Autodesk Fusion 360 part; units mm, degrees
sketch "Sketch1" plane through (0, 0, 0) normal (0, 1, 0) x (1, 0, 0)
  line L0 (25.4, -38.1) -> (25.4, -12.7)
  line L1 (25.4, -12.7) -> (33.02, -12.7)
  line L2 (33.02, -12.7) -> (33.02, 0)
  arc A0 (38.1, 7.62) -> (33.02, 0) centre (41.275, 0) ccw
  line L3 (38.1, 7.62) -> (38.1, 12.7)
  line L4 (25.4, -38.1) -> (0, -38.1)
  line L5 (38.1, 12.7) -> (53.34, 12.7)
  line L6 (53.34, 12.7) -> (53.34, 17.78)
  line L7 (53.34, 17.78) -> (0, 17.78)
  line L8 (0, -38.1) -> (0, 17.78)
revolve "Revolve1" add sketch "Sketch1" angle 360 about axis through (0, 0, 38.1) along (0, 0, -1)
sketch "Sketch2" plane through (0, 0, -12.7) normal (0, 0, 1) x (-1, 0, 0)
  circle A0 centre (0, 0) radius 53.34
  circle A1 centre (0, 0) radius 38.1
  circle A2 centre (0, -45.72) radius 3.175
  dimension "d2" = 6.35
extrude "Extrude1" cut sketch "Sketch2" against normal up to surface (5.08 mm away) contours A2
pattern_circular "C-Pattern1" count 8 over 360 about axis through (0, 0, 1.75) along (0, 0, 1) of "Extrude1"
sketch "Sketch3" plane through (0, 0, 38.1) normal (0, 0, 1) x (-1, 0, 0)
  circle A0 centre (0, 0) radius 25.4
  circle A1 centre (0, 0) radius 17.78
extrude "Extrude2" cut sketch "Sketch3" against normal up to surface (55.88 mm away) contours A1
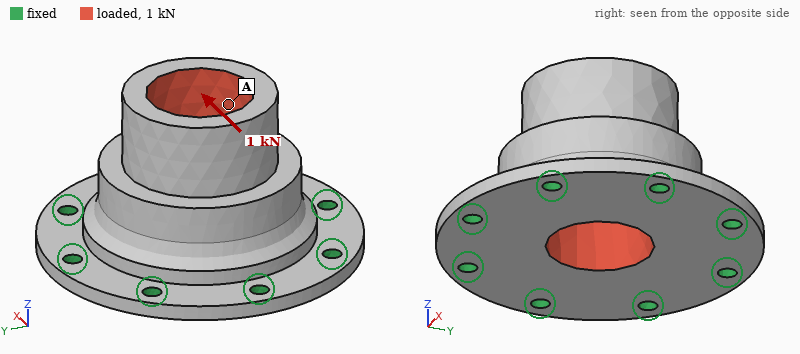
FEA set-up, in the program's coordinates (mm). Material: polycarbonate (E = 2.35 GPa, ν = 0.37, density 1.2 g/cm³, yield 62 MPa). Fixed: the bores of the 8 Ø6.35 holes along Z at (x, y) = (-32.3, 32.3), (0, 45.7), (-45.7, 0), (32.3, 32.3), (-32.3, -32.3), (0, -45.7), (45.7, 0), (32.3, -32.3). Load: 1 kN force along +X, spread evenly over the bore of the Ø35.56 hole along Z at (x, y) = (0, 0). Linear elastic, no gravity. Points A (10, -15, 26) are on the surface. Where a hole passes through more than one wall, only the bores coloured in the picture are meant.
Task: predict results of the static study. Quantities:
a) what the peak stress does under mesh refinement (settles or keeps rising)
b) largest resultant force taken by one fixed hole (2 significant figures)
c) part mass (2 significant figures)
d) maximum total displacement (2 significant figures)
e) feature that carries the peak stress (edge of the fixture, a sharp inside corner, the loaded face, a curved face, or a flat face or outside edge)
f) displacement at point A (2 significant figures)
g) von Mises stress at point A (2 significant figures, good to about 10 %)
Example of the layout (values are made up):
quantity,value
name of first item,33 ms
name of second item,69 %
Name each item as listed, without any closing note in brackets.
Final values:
quantity,value
what the peak stress does under mesh refinement,keeps rising
largest resultant force taken by one fixed hole,240 N
part mass,160 g
maximum total displacement,81 µm
feature that carries the peak stress,edge of the fixture
displacement at point A,60 µm
von Mises stress at point A,0.88 MPa
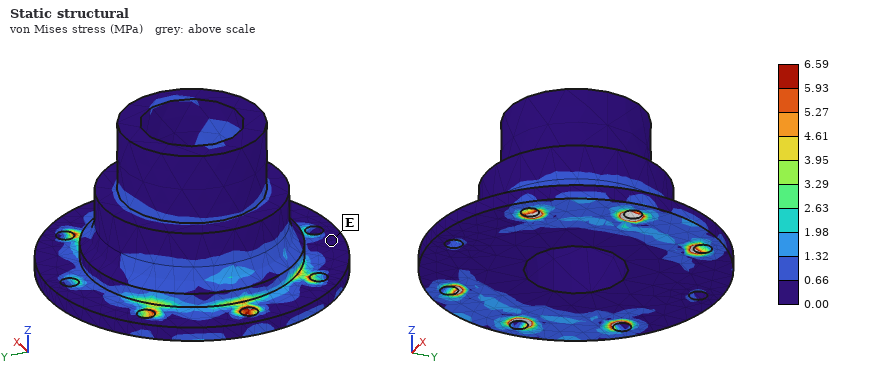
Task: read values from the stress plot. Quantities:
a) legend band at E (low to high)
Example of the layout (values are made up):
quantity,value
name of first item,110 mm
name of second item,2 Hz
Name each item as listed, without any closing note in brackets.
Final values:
quantity,value
legend band at E,0.00 to 0.66 MPa
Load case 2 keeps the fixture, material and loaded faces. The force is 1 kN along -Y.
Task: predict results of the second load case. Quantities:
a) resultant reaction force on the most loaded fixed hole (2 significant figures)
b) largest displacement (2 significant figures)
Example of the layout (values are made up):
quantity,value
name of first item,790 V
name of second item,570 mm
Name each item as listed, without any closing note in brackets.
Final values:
quantity,value
resultant reaction force on the most loaded fixed hole,240 N
largest displacement,81 µm
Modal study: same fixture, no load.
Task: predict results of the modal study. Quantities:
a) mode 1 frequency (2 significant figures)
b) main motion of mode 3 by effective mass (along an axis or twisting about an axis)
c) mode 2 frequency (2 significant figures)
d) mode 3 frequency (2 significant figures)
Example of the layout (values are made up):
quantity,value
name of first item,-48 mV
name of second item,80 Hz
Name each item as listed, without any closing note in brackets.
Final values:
quantity,value
mode 1 frequency,2200 Hz
main motion of mode 3 by effective mass,along Z
mode 2 frequency,2200 Hz
mode 3 frequency,2300 Hz
